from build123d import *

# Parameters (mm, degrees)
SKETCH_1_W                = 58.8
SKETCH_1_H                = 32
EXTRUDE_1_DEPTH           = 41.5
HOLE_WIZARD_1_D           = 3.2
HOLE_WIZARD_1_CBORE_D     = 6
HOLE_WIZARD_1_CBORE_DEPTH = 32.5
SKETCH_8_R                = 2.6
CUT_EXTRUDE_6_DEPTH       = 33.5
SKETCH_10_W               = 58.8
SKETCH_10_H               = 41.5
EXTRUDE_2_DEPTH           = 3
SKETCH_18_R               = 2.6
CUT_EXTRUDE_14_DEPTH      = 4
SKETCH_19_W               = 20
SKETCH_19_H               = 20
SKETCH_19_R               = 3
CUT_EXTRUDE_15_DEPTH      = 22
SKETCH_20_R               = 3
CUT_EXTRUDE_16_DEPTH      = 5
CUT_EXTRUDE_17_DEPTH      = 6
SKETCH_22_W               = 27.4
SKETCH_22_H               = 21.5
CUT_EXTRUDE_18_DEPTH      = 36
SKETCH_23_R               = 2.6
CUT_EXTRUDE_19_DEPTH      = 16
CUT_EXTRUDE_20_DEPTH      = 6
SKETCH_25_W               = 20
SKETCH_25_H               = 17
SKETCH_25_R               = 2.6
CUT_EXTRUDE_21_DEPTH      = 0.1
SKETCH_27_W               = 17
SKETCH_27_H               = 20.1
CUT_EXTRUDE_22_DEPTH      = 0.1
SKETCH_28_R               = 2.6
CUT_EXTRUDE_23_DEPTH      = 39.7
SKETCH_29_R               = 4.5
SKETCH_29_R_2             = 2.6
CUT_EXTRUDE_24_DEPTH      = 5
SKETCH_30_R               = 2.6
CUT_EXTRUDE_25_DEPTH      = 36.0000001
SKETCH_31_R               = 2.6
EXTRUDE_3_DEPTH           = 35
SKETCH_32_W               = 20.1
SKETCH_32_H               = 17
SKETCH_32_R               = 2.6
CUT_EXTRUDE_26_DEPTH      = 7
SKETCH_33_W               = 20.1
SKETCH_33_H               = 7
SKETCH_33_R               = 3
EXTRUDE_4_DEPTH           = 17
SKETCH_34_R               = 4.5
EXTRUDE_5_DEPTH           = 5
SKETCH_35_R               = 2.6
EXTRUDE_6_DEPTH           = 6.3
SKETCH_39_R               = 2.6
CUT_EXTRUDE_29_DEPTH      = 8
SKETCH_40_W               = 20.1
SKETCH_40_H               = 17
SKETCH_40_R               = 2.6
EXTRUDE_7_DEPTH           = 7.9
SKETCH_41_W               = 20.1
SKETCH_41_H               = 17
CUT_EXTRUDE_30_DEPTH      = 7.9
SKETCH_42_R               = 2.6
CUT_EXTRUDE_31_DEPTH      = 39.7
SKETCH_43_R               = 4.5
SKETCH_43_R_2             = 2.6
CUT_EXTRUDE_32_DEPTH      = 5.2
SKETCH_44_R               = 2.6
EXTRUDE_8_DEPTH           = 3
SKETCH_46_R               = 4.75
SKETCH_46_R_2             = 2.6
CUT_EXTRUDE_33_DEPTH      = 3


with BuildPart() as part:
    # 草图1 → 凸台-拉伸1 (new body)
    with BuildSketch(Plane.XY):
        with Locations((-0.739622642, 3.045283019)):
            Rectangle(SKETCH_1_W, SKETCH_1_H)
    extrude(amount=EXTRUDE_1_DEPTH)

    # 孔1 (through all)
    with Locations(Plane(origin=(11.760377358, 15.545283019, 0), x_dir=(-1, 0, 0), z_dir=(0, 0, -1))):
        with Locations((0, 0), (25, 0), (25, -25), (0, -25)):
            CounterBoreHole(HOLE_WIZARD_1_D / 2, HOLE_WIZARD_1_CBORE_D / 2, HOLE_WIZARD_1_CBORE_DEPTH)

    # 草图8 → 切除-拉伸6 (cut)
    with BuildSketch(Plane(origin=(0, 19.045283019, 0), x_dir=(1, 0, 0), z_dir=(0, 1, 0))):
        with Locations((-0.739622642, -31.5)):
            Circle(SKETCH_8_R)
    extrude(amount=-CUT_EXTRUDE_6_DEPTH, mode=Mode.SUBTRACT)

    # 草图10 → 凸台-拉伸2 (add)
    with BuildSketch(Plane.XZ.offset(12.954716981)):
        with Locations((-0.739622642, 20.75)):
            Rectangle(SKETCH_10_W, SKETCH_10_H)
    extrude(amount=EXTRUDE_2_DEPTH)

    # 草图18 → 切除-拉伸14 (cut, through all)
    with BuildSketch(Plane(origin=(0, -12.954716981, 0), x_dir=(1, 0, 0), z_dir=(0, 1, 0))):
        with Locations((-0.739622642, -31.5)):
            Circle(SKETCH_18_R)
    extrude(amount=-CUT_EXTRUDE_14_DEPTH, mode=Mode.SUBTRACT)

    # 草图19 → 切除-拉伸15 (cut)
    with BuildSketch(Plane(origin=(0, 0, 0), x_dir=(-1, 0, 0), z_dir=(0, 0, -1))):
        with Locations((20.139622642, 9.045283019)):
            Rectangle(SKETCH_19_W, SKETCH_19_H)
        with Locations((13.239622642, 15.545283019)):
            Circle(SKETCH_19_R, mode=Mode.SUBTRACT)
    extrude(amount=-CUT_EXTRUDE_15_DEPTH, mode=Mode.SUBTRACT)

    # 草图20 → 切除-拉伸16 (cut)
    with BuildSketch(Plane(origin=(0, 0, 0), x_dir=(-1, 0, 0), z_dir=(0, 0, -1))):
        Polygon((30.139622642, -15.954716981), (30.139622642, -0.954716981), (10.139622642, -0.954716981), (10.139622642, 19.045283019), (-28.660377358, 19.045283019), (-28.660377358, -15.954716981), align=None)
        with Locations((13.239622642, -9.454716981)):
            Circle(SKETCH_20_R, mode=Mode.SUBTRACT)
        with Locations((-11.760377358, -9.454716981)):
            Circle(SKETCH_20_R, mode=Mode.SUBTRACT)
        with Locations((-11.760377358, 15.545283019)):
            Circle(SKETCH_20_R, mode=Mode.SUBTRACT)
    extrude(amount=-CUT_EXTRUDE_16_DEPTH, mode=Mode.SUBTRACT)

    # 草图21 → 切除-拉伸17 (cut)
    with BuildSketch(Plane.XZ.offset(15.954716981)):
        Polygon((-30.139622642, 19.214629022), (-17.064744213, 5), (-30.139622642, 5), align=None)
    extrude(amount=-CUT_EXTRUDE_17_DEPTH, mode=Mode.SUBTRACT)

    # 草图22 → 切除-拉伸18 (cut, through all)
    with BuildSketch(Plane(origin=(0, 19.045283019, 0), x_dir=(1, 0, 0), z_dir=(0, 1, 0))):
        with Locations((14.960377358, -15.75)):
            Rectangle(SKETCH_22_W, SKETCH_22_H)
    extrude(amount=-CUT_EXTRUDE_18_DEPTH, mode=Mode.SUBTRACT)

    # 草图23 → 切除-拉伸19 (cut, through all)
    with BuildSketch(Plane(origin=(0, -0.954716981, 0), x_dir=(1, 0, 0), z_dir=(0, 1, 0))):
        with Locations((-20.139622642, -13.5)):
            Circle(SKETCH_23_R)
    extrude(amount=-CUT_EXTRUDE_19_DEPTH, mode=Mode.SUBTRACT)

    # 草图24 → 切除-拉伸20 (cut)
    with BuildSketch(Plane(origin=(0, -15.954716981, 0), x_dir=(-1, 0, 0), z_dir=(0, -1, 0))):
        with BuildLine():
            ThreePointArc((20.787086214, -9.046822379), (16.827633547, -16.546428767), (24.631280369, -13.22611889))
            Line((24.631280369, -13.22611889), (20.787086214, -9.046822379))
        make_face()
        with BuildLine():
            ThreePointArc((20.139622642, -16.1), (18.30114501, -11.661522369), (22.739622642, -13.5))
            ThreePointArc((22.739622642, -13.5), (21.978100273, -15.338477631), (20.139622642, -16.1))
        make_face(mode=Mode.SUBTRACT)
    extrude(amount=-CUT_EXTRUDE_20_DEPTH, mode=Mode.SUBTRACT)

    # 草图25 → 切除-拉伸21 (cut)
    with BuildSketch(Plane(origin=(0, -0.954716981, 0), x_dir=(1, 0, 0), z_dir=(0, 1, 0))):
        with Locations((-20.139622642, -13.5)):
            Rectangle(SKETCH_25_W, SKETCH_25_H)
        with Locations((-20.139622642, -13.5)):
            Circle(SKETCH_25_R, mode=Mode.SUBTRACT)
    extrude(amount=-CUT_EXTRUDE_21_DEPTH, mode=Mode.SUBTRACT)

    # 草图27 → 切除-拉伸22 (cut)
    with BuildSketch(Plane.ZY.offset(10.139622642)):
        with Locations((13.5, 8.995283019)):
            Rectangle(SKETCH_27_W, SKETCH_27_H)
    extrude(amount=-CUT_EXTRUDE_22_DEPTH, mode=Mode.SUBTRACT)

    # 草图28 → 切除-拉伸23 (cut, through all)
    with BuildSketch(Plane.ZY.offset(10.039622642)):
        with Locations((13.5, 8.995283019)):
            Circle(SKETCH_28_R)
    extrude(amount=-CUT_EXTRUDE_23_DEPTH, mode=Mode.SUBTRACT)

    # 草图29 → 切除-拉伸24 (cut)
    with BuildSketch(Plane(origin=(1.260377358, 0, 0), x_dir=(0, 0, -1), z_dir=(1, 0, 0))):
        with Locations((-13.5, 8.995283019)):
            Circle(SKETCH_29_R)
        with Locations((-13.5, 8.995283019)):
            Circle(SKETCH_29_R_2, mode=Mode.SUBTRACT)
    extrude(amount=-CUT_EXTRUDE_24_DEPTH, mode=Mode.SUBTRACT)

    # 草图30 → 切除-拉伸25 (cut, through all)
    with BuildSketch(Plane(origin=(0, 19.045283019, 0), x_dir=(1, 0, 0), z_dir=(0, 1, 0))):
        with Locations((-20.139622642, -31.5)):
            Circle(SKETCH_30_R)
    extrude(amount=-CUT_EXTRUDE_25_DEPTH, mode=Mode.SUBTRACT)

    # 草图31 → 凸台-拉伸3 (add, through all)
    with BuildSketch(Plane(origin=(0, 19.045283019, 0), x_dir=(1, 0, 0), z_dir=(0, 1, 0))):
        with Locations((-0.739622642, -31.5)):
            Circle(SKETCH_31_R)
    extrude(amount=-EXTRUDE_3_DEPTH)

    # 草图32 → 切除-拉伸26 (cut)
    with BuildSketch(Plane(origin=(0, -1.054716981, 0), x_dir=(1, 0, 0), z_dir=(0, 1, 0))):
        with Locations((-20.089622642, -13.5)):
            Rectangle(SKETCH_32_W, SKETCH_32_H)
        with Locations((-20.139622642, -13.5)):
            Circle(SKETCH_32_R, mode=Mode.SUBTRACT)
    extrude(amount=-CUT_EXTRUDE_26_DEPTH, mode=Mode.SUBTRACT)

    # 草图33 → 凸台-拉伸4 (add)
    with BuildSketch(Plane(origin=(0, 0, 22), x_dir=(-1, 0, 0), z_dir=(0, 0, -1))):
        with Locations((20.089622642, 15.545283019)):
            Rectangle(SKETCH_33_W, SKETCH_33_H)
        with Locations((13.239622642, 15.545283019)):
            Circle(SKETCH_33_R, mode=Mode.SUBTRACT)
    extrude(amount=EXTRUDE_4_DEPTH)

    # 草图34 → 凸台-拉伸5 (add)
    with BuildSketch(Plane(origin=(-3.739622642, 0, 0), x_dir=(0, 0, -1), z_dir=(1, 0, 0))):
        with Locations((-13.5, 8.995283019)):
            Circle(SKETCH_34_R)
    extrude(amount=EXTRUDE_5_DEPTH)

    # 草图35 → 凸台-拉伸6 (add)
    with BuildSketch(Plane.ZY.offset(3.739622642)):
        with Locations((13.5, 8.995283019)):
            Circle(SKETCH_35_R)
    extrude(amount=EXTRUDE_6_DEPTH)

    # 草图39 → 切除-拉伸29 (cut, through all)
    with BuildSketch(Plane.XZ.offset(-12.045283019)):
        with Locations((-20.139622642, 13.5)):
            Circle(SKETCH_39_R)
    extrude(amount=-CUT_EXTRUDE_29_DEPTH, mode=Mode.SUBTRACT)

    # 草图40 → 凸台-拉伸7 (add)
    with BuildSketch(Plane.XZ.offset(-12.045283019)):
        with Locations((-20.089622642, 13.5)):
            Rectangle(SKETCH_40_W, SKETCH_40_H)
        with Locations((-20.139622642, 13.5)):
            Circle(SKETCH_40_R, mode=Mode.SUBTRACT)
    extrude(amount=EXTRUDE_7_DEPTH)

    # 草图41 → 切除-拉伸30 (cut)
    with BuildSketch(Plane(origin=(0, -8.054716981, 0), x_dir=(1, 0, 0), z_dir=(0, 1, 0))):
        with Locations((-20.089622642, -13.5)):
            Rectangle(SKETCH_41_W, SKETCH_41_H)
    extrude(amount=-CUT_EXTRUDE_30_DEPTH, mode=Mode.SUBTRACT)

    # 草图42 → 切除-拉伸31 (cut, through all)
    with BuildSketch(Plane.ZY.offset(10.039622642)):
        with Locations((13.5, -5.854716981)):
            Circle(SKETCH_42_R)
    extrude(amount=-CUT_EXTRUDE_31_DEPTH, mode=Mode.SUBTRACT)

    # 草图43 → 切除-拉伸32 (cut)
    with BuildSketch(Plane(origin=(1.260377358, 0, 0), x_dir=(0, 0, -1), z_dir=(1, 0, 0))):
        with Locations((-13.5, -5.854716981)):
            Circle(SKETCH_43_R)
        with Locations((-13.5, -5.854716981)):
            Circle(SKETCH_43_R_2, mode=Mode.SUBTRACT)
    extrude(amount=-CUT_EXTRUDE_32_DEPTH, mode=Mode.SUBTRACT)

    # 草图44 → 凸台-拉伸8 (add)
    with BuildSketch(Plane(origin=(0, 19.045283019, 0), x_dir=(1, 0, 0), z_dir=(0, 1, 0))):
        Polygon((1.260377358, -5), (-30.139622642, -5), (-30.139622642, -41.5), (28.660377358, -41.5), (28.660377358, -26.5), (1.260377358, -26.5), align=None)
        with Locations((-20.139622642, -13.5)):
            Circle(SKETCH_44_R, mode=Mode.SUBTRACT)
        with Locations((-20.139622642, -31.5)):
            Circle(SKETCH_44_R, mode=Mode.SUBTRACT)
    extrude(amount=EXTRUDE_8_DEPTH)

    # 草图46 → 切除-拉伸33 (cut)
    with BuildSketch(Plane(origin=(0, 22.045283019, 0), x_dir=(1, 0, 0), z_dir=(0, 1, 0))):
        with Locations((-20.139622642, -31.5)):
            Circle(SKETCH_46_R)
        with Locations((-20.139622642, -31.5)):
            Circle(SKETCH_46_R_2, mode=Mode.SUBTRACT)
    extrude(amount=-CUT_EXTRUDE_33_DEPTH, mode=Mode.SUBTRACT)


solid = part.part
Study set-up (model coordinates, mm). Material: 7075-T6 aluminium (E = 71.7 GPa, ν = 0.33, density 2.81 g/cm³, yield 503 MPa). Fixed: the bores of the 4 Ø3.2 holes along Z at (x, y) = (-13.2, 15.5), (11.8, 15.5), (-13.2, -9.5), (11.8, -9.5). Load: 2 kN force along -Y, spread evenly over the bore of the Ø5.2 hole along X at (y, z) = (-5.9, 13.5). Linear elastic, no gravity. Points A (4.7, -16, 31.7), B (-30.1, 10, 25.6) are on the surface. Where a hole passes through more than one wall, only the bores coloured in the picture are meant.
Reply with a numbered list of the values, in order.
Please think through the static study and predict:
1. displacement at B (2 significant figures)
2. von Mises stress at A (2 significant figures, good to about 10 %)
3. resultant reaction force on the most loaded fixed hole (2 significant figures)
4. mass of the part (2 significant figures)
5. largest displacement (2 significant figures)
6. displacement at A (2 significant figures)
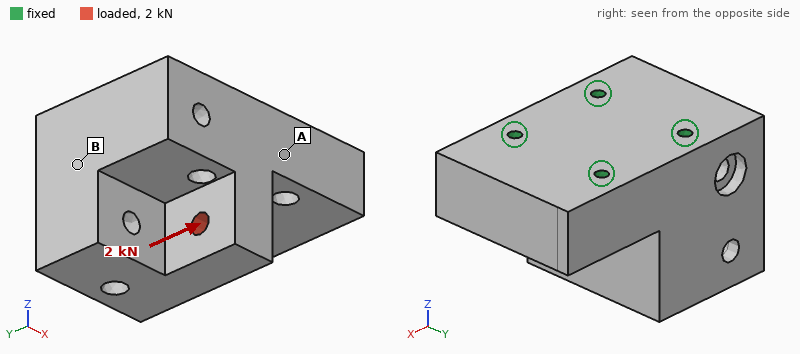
1. 1.8 µm
2. 9.0 MPa
3. 1.3 kN
4. 140 g
5. 11 µm
6. 2.2 µm
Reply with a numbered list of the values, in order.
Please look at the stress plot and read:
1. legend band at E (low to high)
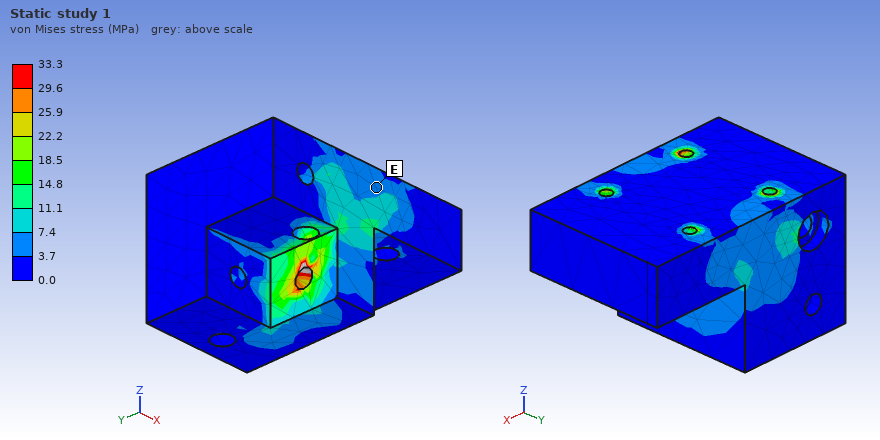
1. 3.7 to 7.4 MPa
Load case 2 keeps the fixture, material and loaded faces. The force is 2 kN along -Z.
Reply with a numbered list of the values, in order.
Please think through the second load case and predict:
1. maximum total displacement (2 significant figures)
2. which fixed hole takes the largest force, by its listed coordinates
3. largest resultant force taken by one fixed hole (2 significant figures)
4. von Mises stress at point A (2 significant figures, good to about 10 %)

1. 6.7 µm
2. (-13.2, -9.5)
3. 1.2 kN
4. 6.6 MPa
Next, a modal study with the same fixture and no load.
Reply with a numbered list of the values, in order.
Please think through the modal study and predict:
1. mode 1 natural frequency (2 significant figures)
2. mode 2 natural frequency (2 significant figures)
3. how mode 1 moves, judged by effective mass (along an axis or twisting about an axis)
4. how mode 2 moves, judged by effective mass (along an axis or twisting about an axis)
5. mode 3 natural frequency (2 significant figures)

1. 11 kHz
2. 13 kHz
3. along X
4. along Y
5. 19 kHz
